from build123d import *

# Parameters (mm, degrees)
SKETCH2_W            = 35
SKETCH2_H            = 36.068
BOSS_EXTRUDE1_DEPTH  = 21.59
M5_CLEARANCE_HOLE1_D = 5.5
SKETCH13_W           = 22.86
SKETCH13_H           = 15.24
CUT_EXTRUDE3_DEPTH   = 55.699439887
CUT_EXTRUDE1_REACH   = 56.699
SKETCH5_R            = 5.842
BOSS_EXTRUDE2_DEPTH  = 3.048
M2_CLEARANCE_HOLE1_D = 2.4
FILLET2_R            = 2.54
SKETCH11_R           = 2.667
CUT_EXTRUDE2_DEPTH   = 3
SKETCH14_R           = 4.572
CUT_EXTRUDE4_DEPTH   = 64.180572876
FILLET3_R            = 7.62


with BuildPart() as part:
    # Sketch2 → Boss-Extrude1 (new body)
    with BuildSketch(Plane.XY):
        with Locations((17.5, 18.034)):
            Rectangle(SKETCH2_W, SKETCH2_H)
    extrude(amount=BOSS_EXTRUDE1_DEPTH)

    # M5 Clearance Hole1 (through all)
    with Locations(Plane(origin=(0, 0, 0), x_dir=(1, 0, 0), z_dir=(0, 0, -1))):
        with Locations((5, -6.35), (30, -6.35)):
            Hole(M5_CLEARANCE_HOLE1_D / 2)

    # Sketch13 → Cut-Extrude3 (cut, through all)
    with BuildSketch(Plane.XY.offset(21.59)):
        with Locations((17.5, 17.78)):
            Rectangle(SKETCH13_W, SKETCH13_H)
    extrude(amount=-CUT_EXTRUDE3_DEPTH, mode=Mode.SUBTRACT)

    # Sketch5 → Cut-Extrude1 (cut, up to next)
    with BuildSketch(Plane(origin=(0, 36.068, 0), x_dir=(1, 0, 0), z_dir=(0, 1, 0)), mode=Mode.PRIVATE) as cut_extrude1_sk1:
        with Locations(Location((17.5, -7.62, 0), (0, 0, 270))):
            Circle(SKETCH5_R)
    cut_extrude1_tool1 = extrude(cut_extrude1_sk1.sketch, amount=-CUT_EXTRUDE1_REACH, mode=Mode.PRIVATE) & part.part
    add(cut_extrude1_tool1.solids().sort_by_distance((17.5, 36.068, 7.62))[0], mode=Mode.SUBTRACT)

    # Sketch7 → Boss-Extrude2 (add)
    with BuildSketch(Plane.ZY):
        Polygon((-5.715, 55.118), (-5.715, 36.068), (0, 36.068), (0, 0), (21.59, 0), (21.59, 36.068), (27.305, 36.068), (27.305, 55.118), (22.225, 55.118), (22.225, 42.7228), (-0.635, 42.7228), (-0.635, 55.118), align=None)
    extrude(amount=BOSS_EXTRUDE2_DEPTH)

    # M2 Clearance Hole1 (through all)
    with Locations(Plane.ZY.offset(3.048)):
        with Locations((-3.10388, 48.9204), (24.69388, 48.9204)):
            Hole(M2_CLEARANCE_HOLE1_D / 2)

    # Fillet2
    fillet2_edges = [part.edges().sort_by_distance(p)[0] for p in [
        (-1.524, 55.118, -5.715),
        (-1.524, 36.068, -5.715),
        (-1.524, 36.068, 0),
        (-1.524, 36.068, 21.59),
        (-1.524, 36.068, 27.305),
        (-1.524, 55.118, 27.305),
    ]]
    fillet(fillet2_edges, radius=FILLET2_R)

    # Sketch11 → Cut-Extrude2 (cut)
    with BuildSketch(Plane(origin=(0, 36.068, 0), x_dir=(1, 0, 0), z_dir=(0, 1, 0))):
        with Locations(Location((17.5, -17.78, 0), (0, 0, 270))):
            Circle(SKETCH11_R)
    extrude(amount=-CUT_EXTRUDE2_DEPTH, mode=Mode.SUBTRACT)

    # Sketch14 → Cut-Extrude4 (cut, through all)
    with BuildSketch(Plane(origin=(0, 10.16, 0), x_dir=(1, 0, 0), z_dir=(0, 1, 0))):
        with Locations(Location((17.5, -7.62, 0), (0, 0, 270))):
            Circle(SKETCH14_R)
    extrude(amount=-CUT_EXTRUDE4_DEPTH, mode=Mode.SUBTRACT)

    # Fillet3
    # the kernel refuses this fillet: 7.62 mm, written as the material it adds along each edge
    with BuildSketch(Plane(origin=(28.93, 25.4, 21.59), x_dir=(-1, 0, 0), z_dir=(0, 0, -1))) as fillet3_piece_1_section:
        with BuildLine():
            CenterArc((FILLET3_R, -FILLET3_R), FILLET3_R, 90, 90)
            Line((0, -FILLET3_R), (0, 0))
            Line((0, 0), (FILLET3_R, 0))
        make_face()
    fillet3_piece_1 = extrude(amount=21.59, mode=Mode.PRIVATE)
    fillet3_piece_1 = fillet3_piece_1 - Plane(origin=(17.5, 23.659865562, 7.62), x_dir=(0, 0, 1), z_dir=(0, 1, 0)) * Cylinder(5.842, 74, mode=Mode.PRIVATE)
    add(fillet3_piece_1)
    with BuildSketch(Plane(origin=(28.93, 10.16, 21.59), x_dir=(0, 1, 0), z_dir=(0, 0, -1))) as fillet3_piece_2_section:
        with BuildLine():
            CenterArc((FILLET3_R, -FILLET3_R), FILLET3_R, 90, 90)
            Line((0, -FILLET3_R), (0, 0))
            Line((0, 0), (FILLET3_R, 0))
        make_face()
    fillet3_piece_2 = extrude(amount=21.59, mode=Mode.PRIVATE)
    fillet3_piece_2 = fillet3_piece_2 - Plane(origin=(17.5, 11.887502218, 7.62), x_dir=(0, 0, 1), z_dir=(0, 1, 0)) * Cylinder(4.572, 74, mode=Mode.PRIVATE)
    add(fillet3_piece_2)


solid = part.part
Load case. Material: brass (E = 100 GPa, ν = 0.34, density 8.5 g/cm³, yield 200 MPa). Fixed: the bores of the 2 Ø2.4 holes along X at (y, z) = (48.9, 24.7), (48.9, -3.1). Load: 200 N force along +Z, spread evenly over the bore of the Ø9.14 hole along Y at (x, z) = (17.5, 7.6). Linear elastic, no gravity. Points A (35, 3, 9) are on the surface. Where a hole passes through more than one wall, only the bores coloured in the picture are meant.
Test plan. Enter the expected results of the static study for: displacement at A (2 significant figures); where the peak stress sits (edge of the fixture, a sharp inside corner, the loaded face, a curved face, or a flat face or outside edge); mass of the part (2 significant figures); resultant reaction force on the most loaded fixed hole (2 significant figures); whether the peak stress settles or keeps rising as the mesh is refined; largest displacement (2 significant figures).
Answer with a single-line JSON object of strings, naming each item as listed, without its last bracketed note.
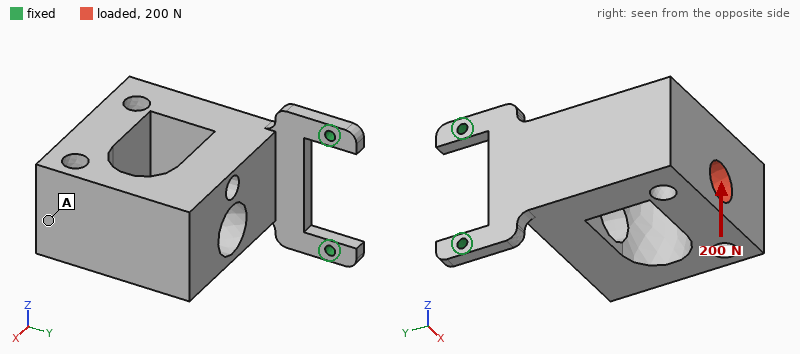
{"displacement at A": "96 µm", "where the peak stress sits": "edge of the fixture", "mass of the part": "180 g", "resultant reaction force on the most loaded fixed hole": "330 N", "whether the peak stress settles or keeps rising as the mesh is refined": "keeps rising", "largest displacement": "100 µm"}
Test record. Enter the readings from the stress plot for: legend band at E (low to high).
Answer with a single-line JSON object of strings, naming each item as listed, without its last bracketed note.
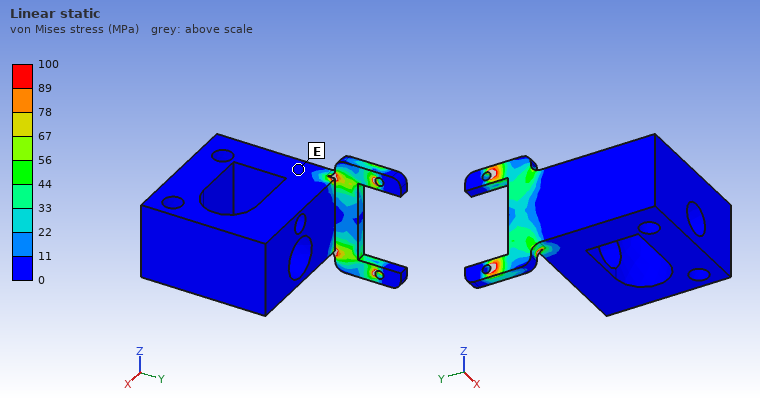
{"legend band at E": "0 to 11 MPa"}
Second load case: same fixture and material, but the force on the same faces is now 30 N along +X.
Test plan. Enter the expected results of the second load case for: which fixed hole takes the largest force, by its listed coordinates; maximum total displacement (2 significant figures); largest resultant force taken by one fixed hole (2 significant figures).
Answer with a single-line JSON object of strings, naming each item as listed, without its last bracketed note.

{"which fixed hole takes the largest force, by its listed coordinates": "(48.9, -3.1)", "maximum total displacement": "0.31 mm", "largest resultant force taken by one fixed hole": "18 N"}
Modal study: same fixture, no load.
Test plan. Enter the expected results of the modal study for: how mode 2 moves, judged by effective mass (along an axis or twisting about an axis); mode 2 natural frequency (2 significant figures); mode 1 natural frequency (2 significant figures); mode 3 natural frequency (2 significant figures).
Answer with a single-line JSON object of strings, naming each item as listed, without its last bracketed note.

{"how mode 2 moves, judged by effective mass": "along Z", "mode 2 natural frequency": "700 Hz", "mode 1 natural frequency": "160 Hz", "mode 3 natural frequency": "1700 Hz"}
